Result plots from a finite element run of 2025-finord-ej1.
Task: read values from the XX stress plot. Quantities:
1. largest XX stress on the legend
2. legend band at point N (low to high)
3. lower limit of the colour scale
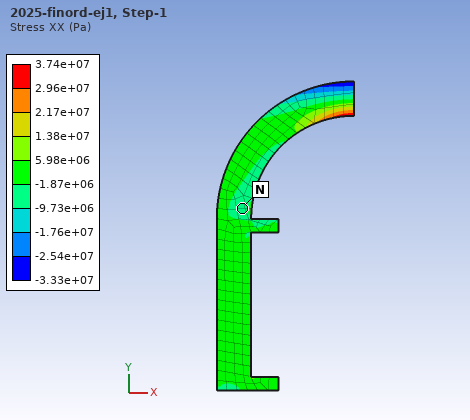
3.74e+07 Pa
-9.73e+06 to -1.87e+06 Pa
-3.33e+07 Pa
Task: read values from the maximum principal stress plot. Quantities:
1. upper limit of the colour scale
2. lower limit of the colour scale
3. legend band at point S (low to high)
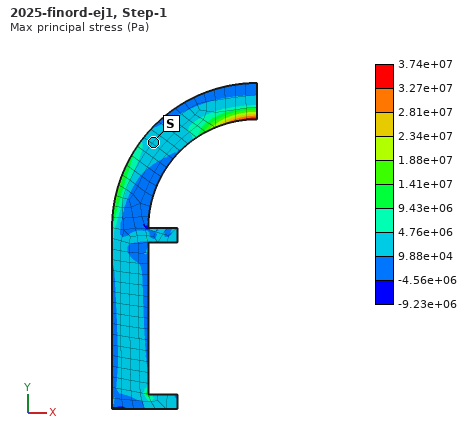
3.74e+07 Pa
-9.23e+06 Pa
9.88e+04 to 4.76e+06 Pa
